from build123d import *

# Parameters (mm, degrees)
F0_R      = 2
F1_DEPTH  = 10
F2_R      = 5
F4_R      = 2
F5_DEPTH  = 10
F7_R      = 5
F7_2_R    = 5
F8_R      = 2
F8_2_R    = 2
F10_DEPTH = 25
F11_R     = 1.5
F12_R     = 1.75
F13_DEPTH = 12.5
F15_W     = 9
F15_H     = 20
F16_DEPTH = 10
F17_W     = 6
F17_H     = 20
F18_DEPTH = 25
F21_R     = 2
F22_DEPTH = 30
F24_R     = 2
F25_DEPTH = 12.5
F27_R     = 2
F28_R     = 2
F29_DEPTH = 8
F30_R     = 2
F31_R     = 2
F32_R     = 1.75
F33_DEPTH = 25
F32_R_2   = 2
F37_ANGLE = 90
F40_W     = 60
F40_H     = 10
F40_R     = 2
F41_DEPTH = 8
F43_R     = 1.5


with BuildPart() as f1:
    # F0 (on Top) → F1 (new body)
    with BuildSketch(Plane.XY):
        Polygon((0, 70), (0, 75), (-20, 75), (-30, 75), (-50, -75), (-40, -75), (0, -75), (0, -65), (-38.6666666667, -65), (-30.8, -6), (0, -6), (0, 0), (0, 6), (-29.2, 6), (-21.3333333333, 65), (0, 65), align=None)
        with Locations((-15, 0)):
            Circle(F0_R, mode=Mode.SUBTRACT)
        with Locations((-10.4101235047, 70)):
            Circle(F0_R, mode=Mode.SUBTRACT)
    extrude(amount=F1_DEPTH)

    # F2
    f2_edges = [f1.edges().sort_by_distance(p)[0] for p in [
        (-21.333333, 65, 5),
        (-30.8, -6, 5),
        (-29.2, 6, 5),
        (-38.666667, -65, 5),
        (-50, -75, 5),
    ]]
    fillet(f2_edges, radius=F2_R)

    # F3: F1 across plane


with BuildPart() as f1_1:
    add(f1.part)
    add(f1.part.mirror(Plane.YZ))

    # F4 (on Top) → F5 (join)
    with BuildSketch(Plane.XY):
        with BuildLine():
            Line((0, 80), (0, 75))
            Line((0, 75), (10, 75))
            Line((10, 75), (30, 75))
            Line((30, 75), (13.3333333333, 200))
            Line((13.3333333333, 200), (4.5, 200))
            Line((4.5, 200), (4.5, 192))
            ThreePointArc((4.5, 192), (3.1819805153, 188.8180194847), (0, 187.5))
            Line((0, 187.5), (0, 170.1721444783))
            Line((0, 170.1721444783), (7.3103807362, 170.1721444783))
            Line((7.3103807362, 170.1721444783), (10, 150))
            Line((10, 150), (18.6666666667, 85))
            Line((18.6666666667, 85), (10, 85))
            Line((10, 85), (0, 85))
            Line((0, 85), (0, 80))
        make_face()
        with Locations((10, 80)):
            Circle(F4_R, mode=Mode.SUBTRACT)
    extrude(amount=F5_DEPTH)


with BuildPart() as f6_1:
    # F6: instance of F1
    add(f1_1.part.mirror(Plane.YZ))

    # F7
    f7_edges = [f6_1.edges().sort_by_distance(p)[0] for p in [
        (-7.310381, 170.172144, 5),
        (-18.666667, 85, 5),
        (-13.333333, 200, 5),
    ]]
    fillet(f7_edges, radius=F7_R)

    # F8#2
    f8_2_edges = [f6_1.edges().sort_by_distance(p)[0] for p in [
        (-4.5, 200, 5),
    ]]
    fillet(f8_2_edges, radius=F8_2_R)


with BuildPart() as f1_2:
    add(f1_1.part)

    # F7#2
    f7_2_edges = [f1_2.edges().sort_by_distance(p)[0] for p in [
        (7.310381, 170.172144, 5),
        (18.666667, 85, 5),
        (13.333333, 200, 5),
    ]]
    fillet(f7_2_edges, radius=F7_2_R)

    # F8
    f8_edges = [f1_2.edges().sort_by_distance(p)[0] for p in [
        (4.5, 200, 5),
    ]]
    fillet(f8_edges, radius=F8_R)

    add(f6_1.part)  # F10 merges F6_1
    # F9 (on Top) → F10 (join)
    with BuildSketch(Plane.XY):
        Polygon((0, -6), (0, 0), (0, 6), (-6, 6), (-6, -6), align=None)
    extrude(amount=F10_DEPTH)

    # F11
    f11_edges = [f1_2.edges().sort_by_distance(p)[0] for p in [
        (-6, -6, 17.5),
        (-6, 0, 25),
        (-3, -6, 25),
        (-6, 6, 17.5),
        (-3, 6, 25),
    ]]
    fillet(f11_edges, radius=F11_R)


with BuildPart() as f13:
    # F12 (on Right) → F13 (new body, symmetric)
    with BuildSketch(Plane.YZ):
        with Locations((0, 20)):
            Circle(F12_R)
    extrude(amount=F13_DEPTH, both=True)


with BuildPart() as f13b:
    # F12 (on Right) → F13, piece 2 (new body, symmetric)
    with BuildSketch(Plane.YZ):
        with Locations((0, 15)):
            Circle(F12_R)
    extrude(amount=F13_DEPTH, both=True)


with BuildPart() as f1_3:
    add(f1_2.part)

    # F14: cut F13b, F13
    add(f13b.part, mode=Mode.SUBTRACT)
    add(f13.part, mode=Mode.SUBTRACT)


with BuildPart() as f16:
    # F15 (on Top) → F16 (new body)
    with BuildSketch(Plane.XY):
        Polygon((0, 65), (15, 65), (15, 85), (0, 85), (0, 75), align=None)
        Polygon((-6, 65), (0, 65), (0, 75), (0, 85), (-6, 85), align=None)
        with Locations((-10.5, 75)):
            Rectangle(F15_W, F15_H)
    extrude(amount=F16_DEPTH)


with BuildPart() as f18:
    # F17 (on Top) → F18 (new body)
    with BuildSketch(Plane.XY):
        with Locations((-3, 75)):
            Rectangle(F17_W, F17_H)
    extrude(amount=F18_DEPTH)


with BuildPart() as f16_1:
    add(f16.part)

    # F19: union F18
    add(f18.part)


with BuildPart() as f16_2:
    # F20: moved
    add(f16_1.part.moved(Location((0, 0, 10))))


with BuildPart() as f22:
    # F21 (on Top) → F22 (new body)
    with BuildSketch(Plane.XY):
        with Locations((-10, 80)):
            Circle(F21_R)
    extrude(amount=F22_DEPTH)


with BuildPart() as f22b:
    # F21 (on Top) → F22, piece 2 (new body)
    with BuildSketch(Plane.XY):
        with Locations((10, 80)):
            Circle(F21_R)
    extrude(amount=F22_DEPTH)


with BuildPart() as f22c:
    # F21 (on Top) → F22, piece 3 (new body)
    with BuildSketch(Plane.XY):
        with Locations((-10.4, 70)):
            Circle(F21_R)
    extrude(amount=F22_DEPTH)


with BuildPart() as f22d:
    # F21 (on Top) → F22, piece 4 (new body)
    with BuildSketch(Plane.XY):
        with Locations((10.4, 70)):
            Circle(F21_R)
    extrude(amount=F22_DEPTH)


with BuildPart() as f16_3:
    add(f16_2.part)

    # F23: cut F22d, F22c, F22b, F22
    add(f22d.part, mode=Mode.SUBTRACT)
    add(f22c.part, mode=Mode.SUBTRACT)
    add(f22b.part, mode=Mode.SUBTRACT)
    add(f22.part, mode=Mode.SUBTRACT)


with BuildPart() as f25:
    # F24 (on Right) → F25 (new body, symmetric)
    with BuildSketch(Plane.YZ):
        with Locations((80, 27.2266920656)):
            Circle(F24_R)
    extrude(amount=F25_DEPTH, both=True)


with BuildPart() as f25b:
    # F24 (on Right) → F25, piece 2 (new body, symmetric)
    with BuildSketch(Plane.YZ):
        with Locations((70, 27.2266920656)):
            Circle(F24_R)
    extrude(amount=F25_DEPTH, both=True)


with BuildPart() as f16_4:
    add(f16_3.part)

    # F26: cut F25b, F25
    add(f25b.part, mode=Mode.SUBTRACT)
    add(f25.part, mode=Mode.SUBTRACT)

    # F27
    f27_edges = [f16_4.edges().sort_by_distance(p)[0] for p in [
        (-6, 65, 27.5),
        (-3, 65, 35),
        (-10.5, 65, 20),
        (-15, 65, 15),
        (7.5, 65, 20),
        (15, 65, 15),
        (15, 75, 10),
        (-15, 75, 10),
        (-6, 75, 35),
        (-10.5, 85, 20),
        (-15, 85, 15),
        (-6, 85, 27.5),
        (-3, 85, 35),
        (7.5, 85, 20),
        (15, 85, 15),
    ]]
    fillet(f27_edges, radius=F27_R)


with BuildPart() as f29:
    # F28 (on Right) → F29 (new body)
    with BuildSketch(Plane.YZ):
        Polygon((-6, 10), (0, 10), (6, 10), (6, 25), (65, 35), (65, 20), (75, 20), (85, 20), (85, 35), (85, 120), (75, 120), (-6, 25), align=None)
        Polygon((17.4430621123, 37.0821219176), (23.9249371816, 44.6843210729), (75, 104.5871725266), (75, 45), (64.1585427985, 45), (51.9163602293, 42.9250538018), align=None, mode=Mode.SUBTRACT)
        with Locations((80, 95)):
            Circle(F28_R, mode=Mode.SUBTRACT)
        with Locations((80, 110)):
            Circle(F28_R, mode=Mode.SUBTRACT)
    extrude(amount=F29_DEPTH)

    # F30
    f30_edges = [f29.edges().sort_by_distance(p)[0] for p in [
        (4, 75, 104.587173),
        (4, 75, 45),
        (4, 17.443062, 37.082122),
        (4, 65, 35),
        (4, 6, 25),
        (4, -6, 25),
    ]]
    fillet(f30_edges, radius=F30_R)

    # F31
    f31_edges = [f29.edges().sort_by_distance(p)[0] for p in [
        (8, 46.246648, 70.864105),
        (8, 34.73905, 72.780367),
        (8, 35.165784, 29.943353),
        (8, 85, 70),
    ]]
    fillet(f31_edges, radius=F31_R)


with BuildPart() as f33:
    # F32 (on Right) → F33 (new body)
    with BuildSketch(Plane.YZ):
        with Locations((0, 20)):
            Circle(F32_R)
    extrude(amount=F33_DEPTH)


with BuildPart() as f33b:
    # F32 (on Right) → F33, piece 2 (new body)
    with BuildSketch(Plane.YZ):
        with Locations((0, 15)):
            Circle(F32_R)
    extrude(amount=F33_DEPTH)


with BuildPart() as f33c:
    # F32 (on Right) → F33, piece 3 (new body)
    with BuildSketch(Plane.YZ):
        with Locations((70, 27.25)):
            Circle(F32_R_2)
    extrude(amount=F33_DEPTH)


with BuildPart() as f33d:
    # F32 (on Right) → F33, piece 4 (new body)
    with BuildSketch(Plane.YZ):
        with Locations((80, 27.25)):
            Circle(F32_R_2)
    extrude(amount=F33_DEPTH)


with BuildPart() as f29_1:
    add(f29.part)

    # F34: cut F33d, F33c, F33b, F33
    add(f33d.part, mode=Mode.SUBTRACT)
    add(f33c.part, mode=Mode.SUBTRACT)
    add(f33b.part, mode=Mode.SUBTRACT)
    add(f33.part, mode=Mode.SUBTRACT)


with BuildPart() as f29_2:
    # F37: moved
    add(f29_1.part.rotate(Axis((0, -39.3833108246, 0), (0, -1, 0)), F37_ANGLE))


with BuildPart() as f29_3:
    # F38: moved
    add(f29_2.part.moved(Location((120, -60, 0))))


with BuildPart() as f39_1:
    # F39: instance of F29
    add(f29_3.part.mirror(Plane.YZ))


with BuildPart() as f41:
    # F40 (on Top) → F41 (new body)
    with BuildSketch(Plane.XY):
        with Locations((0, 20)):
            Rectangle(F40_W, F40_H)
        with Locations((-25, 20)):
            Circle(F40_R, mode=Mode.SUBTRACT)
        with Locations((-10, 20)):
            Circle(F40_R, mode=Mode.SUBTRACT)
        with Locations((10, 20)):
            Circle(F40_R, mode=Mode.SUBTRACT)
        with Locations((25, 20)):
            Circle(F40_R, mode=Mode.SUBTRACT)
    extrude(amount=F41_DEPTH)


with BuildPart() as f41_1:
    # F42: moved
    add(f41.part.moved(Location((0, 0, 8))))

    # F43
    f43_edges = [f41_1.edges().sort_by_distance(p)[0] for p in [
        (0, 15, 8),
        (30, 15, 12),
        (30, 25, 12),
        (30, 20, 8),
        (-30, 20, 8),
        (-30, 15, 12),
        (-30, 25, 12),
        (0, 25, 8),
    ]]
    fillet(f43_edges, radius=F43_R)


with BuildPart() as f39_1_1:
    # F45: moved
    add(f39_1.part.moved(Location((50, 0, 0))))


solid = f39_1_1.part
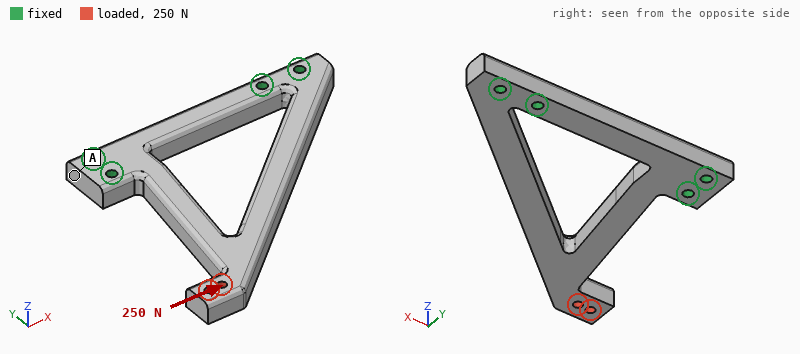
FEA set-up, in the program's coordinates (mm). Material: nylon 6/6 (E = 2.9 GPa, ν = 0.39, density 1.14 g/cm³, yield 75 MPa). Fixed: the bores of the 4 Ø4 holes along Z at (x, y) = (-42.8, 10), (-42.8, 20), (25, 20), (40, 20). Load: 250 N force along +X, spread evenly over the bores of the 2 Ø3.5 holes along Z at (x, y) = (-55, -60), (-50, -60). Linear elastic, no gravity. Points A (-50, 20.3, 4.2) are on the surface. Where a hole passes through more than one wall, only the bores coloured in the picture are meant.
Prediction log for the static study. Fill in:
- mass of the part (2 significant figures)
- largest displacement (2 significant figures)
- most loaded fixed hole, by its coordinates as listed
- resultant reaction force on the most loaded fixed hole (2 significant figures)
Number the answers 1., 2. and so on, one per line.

1. 27 g
2. 0.83 mm
3. (40, 20)
4. 390 N
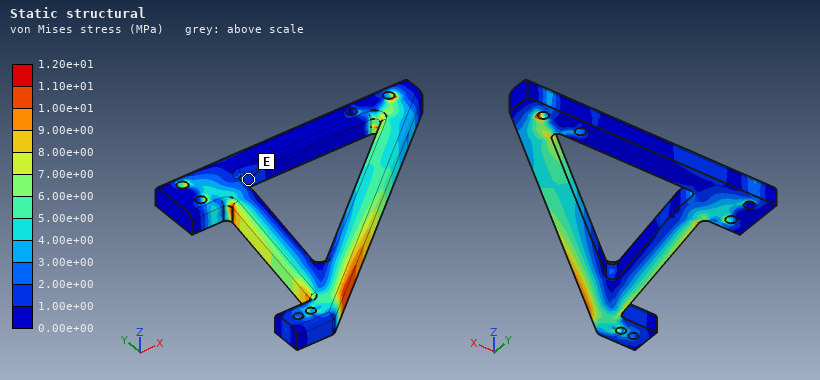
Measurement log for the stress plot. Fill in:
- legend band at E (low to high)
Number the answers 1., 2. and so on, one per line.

1. 1.00e+00 to 2.00e+00 MPa
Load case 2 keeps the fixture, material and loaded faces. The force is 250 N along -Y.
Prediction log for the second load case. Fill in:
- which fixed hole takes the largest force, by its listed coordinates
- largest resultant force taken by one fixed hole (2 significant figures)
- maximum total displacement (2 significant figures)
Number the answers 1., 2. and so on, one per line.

1. (-42.8, 10)
2. 420 N
3. 1.1 mm
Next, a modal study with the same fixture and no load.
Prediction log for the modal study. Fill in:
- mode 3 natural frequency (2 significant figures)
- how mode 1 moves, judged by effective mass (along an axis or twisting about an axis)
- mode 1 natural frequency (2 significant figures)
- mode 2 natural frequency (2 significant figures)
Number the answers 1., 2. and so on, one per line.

1. 1300 Hz
2. along Z
3. 260 Hz
4. 860 Hz
